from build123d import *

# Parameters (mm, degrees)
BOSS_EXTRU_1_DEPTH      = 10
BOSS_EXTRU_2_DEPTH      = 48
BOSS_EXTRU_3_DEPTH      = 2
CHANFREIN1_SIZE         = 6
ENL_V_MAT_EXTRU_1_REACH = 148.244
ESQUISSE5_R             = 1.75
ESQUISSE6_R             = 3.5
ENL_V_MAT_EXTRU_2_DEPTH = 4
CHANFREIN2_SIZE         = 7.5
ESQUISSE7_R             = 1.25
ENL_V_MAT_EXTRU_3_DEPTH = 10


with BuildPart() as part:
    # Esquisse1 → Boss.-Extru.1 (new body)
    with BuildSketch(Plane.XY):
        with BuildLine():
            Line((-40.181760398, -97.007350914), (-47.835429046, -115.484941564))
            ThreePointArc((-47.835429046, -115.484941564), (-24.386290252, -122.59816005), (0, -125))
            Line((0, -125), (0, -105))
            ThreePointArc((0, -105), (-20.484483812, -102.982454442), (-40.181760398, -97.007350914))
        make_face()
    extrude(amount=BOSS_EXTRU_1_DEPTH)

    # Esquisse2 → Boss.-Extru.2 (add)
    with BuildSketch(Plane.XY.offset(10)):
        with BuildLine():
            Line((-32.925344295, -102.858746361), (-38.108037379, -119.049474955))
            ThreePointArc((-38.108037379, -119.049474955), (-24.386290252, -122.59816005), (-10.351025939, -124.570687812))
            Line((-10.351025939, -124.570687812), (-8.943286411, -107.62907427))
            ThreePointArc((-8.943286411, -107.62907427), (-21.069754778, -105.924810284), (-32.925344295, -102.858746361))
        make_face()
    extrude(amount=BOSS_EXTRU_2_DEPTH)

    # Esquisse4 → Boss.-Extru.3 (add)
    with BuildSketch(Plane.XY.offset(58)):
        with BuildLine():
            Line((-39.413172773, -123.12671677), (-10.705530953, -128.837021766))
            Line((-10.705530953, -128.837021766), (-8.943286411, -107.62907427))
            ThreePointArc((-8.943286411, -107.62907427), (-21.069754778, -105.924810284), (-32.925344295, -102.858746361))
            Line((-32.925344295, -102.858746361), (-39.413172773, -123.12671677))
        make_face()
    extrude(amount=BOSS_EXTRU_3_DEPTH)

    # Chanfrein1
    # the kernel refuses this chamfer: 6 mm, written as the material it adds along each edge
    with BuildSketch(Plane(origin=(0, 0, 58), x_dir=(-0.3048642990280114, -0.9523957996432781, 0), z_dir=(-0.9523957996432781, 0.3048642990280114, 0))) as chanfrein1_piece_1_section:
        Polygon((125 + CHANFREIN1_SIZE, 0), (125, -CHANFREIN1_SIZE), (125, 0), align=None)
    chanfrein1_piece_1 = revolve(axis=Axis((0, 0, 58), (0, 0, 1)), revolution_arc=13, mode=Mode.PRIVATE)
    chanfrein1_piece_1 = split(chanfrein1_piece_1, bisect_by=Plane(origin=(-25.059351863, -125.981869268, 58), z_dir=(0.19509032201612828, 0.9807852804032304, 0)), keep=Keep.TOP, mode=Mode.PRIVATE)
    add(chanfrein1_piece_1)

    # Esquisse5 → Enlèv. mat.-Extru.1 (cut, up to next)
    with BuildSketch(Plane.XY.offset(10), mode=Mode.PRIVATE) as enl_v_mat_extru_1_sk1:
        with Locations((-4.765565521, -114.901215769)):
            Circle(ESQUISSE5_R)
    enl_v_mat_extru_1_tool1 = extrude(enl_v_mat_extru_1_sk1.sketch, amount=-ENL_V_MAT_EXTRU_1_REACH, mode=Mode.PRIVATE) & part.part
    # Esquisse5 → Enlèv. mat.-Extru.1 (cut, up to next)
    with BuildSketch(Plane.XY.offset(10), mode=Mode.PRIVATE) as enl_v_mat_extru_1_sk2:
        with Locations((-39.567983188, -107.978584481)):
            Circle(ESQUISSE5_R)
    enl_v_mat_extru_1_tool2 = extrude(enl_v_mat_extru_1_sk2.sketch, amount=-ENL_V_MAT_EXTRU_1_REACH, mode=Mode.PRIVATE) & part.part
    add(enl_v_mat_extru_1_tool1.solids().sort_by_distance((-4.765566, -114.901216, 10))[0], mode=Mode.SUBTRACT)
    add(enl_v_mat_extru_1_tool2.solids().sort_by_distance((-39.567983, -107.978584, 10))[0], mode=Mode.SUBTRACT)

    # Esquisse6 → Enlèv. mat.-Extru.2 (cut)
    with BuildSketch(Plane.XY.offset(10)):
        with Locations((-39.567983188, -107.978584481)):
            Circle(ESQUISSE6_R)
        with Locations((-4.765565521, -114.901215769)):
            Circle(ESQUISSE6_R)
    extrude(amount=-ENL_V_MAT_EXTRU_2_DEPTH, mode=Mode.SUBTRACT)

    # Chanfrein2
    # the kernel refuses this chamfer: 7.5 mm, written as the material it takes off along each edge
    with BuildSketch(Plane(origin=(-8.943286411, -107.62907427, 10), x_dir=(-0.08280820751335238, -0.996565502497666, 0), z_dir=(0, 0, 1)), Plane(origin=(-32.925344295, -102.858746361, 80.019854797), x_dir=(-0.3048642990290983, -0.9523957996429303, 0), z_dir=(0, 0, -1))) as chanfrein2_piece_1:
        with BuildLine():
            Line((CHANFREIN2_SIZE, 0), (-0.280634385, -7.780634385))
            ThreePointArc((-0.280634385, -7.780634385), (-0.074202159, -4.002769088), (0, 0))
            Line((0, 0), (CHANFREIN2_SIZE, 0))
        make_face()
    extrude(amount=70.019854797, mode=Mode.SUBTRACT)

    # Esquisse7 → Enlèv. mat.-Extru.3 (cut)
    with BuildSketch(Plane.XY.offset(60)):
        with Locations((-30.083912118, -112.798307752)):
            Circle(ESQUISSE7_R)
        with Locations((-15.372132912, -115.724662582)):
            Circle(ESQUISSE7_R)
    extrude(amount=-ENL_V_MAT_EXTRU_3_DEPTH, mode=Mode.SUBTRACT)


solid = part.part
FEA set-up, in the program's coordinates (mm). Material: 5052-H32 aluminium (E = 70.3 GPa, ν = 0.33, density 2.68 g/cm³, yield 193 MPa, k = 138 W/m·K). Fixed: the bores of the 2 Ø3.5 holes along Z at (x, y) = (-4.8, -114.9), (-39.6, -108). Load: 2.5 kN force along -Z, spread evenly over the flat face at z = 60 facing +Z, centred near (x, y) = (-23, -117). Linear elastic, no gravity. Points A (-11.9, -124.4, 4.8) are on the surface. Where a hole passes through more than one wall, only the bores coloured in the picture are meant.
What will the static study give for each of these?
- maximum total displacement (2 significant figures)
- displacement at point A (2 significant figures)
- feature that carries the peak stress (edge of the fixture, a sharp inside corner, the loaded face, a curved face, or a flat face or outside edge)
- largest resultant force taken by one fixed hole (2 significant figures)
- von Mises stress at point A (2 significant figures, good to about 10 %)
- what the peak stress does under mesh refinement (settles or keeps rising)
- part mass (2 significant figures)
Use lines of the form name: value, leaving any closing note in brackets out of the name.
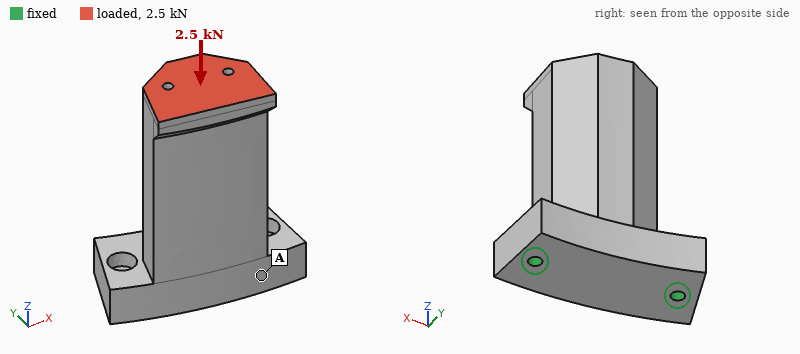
maximum total displacement: 87 µm
displacement at point A: 17 µm
feature that carries the peak stress: edge of the fixture
largest resultant force taken by one fixed hole: 1.4 kN
von Mises stress at point A: 16 MPa
what the peak stress does under mesh refinement: keeps rising
part mass: 77 g
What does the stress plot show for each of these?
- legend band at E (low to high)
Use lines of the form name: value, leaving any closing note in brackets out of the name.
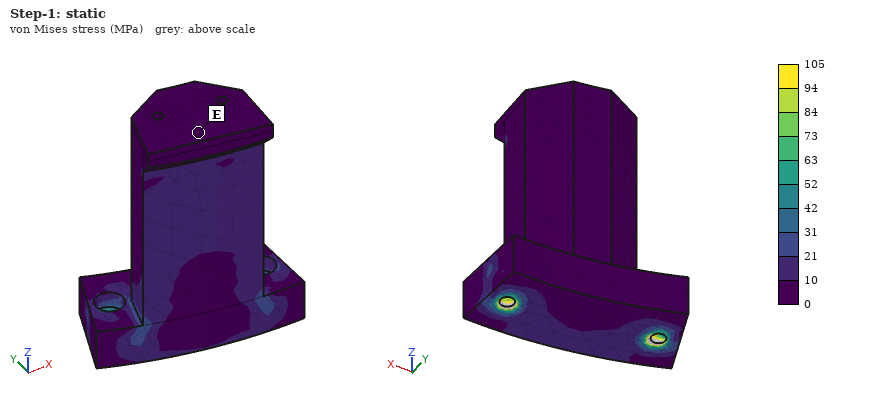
legend band at E: 0 to 10 MPa
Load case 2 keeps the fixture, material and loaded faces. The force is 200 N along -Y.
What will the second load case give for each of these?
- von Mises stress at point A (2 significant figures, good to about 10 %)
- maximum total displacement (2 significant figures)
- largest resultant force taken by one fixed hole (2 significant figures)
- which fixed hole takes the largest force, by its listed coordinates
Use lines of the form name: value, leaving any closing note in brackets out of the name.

von Mises stress at point A: 12 MPa
maximum total displacement: 80 µm
largest resultant force taken by one fixed hole: 140 N
which fixed hole takes the largest force, by its listed coordinates: (-39.6, -108)
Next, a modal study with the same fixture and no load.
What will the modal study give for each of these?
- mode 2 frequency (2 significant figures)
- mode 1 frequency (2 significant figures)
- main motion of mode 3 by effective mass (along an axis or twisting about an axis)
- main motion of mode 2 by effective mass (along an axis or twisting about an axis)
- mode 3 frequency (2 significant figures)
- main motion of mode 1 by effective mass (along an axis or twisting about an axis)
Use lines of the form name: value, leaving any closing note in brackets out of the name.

mode 2 frequency: 4600 Hz
mode 1 frequency: 1800 Hz
main motion of mode 3 by effective mass: along Z
main motion of mode 2 by effective mass: along X
mode 3 frequency: 11 kHz
main motion of mode 1 by effective mass: along Y
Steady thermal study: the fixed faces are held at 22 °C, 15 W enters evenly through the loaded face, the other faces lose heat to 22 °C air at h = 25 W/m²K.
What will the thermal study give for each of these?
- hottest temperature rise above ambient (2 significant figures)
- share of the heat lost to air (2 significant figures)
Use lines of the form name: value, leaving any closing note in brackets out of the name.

hottest temperature rise above ambient: 18 K
share of the heat lost to air: 8.9 %
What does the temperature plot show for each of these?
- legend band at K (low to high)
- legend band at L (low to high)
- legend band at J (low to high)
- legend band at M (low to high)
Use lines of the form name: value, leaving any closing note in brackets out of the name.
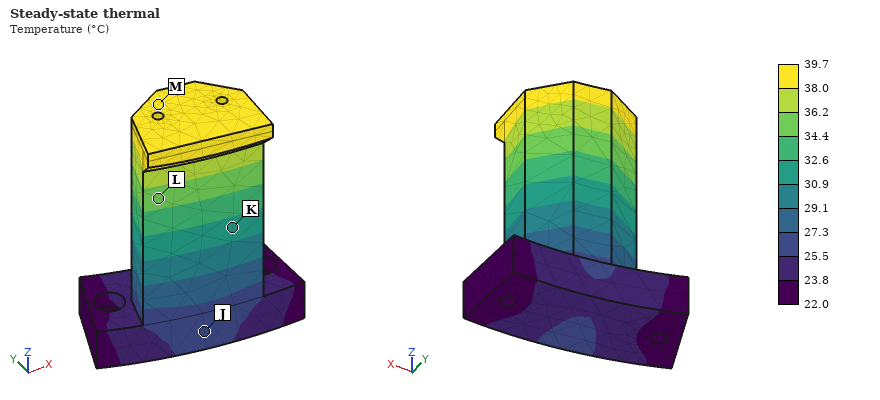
legend band at K: 30.9 to 32.6 °C
legend band at L: 34.4 to 36.2 °C
legend band at J: 25.5 to 27.3 °C
legend band at M: 38.0 to 39.7 °C
